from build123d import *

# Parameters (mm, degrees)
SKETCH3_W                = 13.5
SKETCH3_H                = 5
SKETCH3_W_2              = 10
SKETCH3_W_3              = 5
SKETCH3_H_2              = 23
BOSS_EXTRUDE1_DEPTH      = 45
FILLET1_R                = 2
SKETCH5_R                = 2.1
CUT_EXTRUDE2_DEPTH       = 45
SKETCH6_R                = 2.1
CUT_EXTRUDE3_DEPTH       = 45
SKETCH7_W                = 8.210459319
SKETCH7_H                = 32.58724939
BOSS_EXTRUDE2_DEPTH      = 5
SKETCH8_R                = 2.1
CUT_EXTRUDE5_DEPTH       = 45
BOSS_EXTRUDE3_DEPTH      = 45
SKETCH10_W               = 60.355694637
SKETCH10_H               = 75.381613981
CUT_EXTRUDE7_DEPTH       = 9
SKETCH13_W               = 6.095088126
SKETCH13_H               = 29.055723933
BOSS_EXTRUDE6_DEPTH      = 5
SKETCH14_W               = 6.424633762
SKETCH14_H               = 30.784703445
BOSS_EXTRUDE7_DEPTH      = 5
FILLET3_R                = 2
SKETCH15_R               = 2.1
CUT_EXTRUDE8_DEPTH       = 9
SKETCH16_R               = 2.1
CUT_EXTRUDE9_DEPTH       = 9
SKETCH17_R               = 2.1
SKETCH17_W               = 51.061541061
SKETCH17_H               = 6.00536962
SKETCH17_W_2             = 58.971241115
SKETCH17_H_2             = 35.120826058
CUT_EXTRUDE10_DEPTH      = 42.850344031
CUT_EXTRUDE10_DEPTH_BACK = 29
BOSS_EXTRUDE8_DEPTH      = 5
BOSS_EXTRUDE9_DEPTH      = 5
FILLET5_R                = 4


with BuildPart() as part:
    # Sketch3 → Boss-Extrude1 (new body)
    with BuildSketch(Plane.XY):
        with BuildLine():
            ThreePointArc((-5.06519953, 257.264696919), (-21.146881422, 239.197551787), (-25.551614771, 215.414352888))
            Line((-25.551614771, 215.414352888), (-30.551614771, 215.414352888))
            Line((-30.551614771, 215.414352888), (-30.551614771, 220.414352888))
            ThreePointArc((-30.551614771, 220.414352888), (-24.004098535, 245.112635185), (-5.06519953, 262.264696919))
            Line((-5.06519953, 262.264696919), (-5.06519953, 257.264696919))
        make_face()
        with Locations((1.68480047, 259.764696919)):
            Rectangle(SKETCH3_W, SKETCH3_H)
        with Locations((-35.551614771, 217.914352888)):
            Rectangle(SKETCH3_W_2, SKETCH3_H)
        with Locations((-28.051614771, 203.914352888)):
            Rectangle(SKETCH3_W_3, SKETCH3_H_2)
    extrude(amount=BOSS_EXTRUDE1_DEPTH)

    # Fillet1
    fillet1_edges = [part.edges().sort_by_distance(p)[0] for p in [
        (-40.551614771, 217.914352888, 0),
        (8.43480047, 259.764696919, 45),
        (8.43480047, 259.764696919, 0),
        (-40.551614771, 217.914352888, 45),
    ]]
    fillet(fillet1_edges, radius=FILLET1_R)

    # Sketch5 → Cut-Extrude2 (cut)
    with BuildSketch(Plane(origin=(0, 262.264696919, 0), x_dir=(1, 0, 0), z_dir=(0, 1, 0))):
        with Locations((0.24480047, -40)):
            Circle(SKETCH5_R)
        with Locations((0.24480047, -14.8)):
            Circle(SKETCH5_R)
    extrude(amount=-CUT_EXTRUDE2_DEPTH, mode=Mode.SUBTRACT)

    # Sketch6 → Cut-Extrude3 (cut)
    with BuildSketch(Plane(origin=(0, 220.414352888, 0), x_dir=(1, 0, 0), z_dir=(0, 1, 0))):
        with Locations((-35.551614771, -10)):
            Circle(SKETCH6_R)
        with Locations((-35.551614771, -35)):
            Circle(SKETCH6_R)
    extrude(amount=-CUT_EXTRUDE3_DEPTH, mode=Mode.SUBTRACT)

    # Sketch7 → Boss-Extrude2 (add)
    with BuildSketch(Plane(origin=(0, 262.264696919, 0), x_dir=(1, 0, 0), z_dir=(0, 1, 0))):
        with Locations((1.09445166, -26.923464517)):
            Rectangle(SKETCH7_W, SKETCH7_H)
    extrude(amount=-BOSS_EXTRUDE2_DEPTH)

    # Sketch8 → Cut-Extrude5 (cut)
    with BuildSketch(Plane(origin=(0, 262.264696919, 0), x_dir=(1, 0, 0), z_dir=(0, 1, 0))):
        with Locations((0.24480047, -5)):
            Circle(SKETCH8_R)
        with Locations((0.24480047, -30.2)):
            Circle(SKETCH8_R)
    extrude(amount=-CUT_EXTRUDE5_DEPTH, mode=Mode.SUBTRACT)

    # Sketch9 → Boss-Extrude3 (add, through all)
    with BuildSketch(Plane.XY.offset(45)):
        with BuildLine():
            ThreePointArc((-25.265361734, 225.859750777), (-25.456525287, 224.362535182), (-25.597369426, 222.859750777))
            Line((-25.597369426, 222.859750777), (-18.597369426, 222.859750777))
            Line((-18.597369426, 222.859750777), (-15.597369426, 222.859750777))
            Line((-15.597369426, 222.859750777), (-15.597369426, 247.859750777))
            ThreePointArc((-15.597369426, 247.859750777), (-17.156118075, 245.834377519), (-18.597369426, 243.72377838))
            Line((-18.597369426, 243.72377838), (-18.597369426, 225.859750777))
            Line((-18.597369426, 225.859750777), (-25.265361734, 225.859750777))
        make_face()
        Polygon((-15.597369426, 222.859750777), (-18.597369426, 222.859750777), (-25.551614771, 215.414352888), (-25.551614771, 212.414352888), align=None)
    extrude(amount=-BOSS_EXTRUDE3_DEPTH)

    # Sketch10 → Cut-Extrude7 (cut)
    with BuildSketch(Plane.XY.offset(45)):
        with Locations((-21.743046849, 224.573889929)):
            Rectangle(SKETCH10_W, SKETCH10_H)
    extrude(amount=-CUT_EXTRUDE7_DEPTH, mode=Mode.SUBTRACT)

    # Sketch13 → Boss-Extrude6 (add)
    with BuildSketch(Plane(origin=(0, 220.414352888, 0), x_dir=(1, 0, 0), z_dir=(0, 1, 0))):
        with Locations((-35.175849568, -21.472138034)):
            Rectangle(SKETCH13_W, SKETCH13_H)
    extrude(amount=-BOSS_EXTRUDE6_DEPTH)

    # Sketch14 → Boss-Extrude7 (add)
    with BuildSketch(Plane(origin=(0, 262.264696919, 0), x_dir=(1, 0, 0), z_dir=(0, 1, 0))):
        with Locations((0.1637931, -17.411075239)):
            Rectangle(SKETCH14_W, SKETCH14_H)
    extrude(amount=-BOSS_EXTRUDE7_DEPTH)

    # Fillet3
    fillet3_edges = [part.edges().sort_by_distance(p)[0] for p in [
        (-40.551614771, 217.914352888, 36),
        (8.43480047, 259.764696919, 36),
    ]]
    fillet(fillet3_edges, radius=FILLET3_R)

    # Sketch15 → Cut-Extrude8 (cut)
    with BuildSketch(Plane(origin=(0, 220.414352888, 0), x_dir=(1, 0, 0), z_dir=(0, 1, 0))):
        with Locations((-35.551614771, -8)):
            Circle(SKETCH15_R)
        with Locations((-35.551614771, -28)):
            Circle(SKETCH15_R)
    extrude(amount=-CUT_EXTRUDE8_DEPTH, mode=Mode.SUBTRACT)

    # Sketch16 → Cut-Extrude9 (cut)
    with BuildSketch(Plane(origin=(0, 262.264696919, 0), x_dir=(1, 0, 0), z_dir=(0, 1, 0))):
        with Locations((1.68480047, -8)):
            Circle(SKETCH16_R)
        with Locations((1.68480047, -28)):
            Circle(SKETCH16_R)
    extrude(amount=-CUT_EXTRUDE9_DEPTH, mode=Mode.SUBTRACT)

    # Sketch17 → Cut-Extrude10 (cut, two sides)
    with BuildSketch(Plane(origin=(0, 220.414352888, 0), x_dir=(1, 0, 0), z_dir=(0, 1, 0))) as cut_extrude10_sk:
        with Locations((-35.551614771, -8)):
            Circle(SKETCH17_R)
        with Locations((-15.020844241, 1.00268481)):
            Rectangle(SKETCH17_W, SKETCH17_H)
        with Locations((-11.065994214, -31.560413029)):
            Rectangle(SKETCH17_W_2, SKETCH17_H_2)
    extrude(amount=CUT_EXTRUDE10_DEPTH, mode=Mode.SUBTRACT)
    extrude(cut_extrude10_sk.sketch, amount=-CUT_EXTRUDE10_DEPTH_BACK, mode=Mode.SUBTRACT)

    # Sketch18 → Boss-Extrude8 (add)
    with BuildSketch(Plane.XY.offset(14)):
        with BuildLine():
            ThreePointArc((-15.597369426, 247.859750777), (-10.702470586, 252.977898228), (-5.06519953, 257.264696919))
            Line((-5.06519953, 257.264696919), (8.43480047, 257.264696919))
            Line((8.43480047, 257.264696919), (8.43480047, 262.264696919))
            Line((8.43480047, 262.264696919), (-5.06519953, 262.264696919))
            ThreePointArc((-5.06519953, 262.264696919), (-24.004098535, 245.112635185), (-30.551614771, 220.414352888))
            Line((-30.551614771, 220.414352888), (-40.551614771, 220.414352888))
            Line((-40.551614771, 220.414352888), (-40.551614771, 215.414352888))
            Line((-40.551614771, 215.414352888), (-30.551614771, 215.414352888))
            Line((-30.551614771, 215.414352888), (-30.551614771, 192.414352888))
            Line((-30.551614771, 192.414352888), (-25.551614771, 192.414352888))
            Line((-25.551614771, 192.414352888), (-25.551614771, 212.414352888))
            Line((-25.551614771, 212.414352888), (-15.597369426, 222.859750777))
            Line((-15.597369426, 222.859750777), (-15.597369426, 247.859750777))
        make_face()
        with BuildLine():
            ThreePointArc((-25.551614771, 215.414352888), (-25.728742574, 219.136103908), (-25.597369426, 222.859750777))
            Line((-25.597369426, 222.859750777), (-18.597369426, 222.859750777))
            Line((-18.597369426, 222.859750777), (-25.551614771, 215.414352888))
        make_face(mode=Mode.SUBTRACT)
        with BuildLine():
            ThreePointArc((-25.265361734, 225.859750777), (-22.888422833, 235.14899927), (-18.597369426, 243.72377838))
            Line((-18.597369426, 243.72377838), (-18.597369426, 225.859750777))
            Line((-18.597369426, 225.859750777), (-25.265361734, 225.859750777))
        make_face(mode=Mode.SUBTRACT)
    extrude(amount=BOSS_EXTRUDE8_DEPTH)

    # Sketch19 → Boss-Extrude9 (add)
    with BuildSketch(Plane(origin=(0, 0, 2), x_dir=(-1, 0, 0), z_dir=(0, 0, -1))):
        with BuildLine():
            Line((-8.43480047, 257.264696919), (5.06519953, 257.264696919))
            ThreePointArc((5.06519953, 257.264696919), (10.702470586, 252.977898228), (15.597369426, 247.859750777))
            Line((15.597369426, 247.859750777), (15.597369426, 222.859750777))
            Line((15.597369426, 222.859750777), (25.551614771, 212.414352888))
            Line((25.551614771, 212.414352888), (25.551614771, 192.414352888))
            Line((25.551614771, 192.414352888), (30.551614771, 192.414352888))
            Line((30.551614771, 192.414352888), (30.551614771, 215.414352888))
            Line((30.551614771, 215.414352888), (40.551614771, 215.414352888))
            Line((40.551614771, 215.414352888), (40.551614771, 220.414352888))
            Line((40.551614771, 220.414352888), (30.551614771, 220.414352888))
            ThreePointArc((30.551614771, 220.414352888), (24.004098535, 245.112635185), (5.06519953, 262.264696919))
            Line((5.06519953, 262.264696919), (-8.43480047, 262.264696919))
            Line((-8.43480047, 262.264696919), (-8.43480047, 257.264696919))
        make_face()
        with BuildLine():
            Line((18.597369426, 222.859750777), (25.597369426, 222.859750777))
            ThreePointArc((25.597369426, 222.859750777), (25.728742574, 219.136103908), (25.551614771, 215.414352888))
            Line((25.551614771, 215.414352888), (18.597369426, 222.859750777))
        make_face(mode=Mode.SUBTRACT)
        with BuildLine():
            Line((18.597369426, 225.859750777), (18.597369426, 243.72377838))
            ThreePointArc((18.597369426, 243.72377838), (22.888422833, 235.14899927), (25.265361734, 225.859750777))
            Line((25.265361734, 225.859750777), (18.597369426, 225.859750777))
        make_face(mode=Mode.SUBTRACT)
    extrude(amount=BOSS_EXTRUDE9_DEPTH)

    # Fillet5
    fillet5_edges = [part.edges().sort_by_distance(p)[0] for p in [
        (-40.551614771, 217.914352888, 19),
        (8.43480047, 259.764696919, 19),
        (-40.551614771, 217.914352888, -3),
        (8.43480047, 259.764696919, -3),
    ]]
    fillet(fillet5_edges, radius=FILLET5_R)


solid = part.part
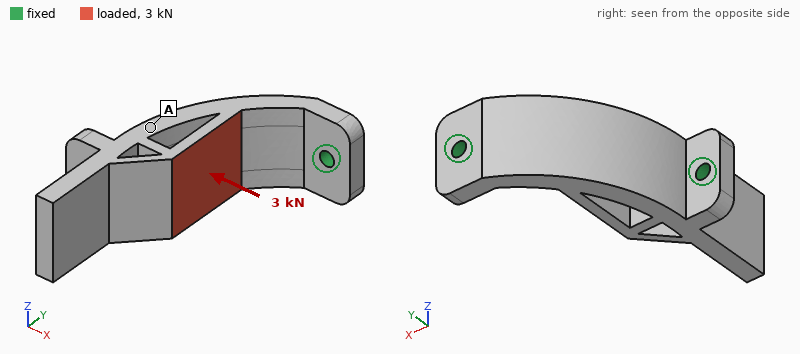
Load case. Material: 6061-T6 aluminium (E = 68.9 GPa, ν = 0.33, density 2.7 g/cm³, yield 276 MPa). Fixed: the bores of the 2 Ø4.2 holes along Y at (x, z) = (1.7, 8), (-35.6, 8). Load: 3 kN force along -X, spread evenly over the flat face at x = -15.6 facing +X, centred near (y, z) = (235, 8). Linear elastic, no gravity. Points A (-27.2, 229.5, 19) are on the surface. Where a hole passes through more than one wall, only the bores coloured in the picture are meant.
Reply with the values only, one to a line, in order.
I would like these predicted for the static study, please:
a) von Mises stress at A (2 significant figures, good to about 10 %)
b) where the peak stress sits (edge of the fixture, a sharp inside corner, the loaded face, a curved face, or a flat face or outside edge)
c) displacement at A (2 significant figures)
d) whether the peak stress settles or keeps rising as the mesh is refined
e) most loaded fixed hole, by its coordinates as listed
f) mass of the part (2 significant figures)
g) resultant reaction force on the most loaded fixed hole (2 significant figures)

16 MPa
edge of the fixture
26 µm
keeps rising
(1.7, 8)
36 g
2.0 kN
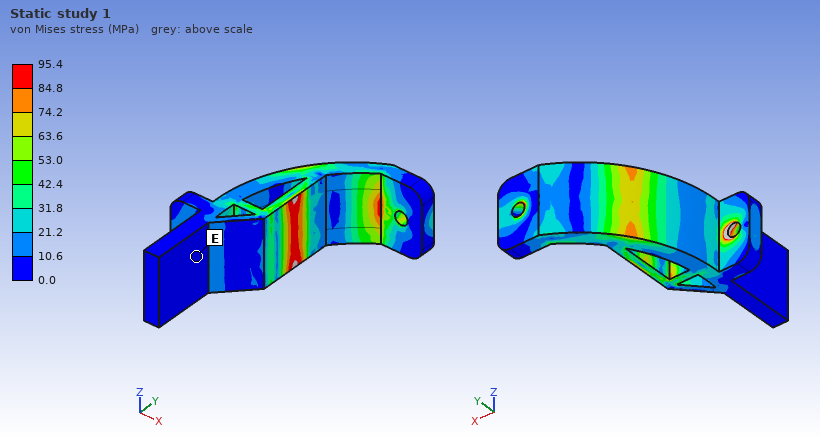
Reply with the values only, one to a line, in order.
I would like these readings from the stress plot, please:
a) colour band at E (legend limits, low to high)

0.0 to 10.6 MPa
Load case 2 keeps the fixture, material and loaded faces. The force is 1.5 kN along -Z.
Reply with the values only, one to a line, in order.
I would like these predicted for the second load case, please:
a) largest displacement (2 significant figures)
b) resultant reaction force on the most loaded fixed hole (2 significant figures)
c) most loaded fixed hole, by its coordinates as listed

38 µm
860 N
(-35.6, 8)
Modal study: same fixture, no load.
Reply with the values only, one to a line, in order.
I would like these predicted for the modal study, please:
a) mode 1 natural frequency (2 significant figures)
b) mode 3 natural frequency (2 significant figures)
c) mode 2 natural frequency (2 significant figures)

6100 Hz
9500 Hz
6800 Hz
